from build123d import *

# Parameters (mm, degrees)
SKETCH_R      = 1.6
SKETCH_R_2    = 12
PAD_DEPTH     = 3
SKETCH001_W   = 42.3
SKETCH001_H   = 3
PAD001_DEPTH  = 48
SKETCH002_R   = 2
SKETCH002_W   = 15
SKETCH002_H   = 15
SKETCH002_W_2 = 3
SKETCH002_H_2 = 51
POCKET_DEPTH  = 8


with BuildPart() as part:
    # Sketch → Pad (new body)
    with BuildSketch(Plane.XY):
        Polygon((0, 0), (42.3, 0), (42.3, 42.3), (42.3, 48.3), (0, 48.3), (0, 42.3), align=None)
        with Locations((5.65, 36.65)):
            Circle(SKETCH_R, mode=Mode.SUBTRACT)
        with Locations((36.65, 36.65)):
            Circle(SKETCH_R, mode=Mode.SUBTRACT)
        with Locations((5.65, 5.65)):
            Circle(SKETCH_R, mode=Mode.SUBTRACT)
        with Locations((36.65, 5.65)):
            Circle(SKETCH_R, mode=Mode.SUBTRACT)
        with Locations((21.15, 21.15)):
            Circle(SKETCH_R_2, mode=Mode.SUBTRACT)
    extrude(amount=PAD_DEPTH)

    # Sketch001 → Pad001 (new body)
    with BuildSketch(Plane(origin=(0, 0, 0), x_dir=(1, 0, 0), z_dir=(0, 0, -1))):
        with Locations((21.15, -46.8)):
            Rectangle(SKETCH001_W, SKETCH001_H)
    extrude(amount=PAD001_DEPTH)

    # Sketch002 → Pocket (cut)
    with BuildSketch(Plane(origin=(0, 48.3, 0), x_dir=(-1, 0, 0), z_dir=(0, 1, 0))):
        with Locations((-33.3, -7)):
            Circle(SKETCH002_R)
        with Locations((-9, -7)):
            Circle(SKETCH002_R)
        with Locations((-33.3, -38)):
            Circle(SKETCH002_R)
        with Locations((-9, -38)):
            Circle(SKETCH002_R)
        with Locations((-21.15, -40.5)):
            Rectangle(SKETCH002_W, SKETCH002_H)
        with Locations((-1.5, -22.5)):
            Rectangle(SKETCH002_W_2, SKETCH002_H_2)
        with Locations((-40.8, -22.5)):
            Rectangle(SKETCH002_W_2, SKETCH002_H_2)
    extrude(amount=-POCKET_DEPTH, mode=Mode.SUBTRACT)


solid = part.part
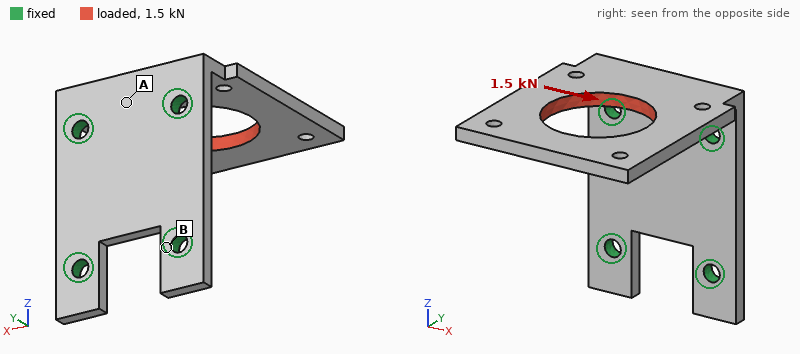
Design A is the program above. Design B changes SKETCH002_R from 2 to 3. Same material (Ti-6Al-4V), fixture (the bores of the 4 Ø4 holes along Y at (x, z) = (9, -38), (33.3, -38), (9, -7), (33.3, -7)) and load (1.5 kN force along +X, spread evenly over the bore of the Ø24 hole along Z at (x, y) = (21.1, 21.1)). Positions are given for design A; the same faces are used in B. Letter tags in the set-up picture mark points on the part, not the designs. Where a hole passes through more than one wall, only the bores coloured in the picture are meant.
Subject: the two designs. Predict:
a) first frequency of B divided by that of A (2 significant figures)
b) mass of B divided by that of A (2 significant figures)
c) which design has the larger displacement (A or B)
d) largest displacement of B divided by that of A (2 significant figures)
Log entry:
1.0
0.98
A
0.77
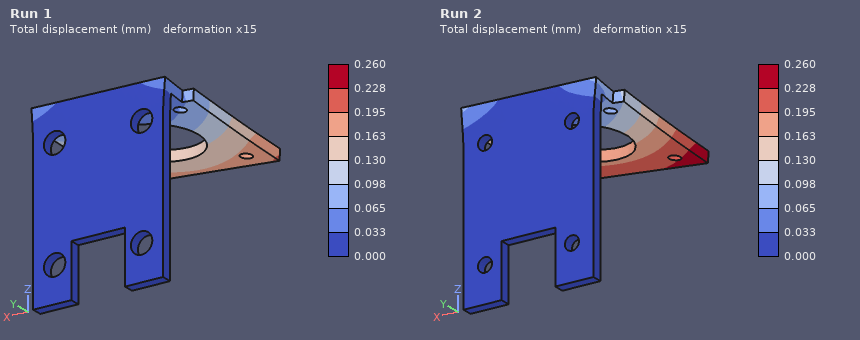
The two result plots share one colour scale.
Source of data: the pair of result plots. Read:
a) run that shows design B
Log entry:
Run 1
